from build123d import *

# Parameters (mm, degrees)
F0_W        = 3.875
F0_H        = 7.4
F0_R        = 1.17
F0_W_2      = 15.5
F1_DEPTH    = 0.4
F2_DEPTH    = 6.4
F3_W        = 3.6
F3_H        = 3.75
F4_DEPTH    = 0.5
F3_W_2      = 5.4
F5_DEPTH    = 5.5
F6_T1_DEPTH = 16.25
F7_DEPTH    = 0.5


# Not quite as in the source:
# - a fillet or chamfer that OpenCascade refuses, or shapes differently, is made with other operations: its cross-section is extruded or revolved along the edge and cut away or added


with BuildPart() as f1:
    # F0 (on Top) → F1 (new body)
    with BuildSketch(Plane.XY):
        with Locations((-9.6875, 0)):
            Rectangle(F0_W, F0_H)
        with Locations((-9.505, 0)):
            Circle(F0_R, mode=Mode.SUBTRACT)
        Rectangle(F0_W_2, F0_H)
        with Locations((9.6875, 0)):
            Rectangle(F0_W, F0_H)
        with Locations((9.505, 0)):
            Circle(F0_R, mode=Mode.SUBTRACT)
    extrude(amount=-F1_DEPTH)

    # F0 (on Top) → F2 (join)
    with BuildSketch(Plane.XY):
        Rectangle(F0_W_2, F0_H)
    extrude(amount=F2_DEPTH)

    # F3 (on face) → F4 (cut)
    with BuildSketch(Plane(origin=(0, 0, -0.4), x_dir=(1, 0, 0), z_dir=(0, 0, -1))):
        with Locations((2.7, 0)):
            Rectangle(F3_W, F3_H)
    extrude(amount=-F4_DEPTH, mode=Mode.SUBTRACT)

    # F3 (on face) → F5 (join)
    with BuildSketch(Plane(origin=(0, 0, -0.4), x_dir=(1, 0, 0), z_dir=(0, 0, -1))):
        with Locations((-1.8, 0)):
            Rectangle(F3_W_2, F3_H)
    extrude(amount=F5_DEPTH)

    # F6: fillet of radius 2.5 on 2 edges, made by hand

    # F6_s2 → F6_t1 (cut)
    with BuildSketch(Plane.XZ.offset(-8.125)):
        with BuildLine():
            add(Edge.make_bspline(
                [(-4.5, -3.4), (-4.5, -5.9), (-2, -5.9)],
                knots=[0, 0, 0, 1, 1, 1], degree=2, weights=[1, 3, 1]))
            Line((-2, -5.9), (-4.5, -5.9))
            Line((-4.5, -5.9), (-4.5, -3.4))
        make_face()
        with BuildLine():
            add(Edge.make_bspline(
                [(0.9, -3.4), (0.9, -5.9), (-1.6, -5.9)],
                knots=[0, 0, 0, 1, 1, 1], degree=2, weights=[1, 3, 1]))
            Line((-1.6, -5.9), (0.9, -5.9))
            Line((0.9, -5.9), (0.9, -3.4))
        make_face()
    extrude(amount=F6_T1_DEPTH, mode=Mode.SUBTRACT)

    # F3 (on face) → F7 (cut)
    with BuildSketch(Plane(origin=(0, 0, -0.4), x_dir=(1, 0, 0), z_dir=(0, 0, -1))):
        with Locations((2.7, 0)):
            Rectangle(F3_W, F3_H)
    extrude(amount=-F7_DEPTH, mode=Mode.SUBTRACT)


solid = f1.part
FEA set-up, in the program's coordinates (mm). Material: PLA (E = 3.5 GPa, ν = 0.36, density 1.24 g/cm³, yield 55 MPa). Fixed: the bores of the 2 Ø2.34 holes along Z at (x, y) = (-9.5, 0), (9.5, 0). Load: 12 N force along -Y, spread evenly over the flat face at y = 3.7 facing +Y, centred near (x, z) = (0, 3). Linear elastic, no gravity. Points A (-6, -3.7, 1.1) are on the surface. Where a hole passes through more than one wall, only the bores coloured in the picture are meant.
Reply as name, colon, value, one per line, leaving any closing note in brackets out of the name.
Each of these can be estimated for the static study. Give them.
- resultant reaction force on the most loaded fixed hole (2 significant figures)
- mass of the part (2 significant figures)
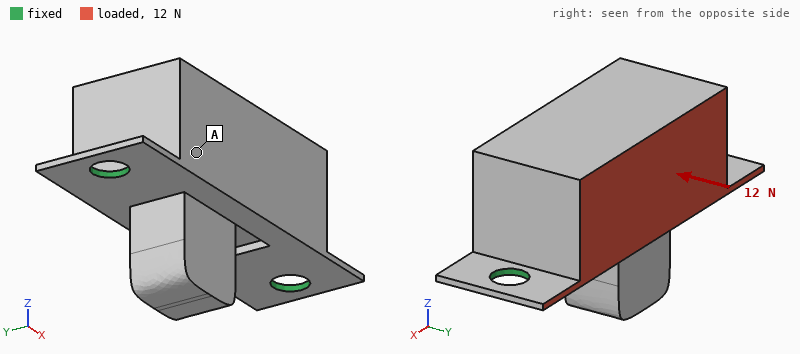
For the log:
resultant reaction force on the most loaded fixed hole: 6.0 N
mass of the part: 1.1 g
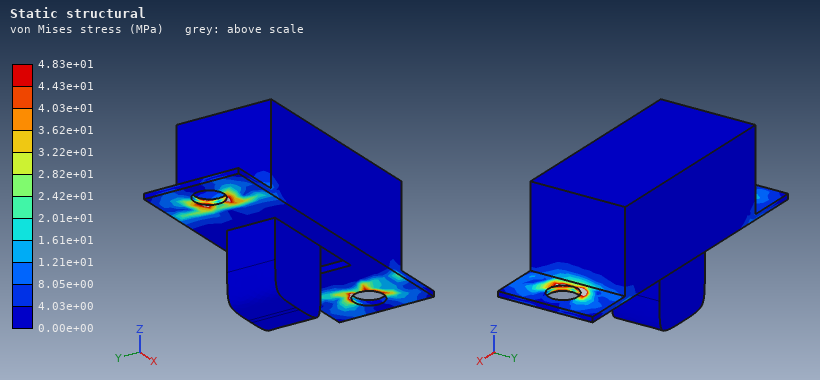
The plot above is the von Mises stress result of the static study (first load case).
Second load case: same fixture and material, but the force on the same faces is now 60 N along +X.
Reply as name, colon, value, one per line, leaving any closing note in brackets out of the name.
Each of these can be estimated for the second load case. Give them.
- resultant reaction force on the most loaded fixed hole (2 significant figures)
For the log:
resultant reaction force on the most loaded fixed hole: 35 N
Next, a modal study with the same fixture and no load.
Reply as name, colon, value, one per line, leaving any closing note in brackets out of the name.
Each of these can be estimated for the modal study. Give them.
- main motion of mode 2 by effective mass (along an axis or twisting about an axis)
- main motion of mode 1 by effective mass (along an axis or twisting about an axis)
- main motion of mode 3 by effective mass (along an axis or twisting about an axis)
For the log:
main motion of mode 2 by effective mass: along Z
main motion of mode 1 by effective mass: along Y
main motion of mode 3 by effective mass: along X
